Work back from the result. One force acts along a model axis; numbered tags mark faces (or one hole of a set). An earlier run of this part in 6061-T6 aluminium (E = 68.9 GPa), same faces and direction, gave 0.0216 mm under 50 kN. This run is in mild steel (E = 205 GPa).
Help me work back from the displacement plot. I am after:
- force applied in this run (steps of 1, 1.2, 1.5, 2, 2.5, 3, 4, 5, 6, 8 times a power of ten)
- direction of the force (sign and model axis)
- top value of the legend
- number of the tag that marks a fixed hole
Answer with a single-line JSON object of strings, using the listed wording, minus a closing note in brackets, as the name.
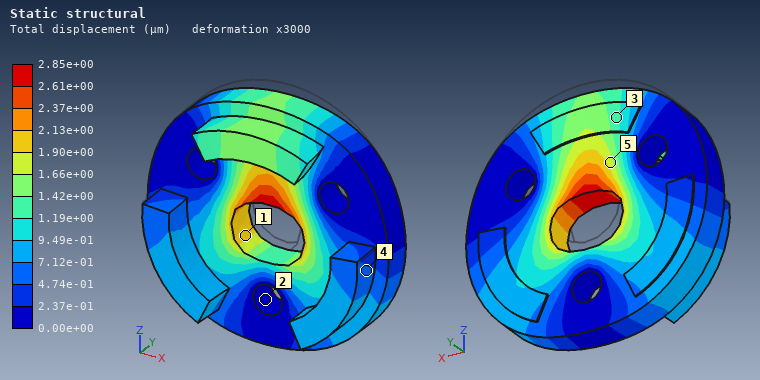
{"force applied in this run": "20 kN", "direction of the force": "-Z", "top value of the legend": "2.85e+00 µm", "number of the tag that marks a fixed hole": "2"}
